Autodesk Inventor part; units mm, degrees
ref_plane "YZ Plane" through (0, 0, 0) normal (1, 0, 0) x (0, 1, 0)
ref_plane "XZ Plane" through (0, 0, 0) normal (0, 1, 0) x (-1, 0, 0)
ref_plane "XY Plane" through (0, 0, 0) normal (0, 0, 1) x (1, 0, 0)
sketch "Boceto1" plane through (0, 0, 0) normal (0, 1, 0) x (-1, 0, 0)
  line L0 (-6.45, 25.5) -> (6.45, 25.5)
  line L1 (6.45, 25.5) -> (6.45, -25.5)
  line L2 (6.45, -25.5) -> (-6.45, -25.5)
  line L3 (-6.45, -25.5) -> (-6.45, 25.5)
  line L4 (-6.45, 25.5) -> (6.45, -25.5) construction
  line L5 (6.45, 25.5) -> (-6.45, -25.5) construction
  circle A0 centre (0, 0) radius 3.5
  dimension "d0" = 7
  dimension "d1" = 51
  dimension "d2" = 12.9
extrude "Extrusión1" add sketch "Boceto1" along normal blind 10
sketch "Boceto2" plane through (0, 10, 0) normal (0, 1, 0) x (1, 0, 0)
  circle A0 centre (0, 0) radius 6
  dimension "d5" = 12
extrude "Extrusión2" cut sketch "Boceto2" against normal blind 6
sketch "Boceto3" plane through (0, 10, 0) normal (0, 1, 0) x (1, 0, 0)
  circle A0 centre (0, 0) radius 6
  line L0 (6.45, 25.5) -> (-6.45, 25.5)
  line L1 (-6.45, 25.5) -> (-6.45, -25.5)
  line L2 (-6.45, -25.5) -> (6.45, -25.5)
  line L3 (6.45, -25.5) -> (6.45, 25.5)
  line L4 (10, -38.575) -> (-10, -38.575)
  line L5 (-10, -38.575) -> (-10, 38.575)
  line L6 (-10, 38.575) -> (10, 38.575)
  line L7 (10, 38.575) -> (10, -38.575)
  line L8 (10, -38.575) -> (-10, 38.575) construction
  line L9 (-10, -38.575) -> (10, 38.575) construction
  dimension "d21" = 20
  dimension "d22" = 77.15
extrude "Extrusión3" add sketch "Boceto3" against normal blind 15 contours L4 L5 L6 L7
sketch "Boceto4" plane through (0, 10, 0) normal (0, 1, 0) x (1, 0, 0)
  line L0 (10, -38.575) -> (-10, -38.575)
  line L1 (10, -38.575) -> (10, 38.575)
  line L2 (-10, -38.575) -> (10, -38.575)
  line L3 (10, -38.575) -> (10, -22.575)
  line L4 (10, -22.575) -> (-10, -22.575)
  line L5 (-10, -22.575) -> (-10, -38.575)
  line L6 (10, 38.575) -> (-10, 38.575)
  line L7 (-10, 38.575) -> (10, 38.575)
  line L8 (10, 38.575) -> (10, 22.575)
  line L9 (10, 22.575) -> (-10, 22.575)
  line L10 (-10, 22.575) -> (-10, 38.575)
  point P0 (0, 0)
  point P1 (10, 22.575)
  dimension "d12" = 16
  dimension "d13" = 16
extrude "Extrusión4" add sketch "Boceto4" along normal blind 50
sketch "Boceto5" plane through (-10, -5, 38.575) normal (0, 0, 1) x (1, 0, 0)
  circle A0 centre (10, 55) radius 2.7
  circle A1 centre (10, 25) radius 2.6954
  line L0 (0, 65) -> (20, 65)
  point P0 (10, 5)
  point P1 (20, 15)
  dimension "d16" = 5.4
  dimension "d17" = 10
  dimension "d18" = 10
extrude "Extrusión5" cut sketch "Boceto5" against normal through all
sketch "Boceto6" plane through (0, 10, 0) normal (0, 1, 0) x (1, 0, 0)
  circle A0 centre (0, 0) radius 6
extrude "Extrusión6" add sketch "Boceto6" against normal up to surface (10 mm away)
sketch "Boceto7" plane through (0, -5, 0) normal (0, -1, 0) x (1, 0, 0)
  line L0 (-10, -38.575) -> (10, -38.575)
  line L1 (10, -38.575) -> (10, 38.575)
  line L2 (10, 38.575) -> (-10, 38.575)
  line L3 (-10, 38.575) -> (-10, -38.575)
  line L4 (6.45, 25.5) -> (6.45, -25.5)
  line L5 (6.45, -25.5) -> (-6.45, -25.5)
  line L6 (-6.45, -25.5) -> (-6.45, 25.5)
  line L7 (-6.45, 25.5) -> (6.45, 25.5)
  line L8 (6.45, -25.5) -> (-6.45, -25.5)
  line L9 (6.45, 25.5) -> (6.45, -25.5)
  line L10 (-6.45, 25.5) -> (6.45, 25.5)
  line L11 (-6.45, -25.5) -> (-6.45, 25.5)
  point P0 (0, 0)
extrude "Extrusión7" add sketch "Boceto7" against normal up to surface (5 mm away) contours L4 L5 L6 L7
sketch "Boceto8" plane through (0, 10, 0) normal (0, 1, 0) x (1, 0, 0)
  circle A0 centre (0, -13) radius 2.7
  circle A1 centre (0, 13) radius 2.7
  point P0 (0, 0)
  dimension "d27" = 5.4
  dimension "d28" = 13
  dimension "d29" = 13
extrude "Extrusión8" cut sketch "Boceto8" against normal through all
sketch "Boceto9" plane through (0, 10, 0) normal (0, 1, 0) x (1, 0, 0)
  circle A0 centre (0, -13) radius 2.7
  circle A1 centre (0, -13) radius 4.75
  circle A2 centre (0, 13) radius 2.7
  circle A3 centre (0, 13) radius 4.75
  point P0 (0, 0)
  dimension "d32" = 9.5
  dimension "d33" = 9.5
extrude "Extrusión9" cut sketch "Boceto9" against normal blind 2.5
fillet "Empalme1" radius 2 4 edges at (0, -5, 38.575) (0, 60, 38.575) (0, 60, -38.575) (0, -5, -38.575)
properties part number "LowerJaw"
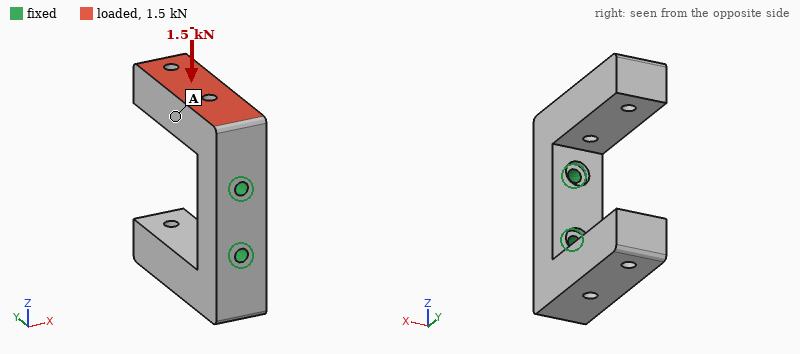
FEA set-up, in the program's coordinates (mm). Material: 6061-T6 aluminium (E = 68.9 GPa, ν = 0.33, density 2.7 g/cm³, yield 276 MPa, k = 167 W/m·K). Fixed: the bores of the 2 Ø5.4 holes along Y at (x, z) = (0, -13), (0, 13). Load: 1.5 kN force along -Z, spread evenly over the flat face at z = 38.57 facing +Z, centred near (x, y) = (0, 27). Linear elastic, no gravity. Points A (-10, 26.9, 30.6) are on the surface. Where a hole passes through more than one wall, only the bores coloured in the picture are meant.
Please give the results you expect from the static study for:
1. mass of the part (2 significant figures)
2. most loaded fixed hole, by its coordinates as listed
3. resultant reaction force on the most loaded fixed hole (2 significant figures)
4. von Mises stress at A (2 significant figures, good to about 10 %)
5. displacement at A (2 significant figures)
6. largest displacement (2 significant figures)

140 g
(0, 13)
1.2 kN
9.8 MPa
0.062 mm
0.17 mm
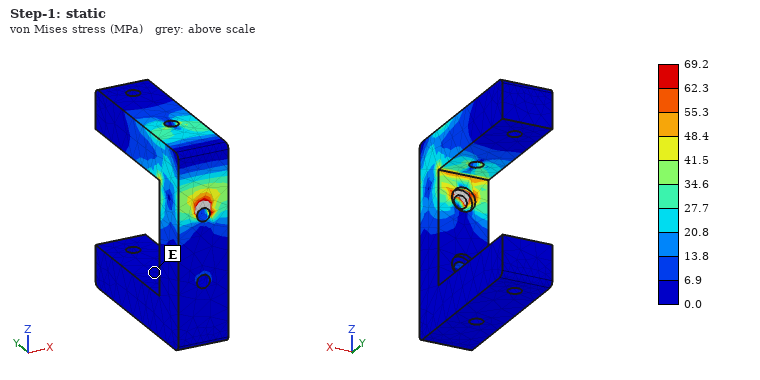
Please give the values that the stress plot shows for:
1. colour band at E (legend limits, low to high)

0.0 to 6.9 MPa
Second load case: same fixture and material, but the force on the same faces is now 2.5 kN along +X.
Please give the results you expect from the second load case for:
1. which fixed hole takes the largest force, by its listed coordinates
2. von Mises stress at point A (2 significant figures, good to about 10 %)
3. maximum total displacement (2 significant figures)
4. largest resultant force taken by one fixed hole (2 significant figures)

(0, 13)
21 MPa
0.28 mm
4.0 kN
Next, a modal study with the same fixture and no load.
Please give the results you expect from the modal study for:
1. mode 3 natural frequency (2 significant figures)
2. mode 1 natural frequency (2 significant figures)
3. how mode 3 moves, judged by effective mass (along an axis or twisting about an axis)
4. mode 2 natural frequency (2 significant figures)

2600 Hz
2400 Hz
along X
2500 Hz
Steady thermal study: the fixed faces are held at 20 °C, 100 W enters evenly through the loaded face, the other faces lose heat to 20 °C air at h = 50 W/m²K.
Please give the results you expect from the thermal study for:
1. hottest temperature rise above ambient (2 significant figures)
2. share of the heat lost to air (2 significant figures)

68 K
11 %
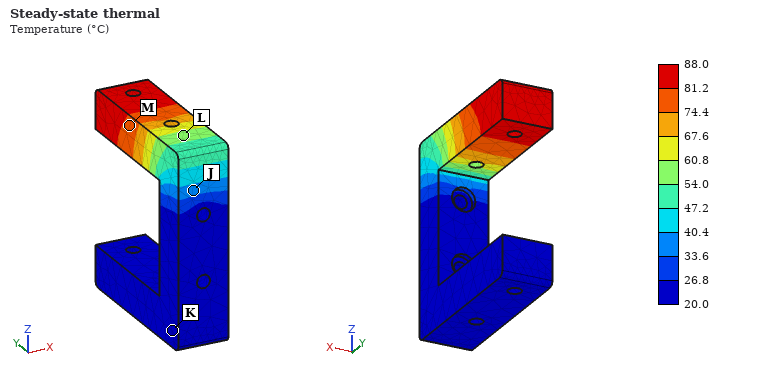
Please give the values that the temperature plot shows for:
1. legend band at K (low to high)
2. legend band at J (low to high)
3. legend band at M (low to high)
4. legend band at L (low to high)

20.0 to 26.8 °C
33.6 to 40.4 °C
74.4 to 81.2 °C
54.0 to 60.8 °C
